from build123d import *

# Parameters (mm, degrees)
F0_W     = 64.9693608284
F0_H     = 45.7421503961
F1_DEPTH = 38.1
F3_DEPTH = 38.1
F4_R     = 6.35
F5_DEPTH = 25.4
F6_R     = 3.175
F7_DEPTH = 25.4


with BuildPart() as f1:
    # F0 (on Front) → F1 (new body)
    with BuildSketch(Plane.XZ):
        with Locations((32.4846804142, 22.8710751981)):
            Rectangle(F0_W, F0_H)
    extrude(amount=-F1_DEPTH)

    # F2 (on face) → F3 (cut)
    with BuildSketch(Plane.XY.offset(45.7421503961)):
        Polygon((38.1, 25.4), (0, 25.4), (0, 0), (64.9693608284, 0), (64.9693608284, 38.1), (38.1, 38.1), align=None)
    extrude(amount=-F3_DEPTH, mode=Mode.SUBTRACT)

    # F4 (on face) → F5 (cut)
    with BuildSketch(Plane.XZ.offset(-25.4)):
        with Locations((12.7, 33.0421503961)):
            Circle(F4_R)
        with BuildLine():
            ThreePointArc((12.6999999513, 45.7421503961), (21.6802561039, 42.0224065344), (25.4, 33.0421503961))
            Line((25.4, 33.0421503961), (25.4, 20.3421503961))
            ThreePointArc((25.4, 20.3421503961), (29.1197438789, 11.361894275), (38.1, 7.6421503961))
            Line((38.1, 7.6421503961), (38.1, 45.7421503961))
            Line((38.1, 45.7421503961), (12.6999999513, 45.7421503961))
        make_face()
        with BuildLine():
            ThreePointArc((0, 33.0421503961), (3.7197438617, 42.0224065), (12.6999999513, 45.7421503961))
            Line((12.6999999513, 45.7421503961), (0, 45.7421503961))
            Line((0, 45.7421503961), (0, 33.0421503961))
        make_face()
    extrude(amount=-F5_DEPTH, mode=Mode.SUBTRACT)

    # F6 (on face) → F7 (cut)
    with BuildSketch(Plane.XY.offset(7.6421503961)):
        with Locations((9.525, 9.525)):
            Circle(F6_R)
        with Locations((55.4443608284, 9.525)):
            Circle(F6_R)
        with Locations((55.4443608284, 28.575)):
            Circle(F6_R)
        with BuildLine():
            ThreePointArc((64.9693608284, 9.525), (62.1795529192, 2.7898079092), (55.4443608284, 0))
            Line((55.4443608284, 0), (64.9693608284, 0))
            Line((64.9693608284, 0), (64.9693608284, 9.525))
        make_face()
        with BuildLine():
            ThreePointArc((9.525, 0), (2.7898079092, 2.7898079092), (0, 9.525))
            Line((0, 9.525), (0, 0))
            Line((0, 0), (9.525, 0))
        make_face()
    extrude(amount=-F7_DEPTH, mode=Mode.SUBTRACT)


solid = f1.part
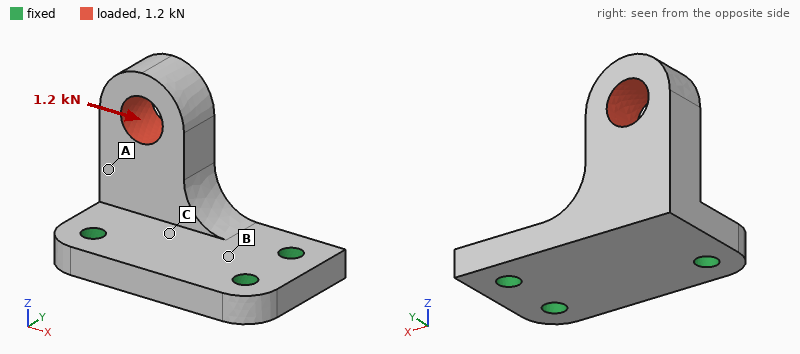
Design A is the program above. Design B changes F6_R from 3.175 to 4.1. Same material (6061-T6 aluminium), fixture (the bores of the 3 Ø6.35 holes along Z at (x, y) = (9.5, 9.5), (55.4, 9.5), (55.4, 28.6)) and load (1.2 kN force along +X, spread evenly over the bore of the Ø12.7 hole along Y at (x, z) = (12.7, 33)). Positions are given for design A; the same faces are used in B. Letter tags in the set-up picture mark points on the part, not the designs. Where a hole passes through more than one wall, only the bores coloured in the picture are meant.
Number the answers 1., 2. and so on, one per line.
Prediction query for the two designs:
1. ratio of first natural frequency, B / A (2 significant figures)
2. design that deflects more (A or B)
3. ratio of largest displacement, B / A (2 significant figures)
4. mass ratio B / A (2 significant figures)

1. 1.0
2. A
3. 0.92
4. 0.98
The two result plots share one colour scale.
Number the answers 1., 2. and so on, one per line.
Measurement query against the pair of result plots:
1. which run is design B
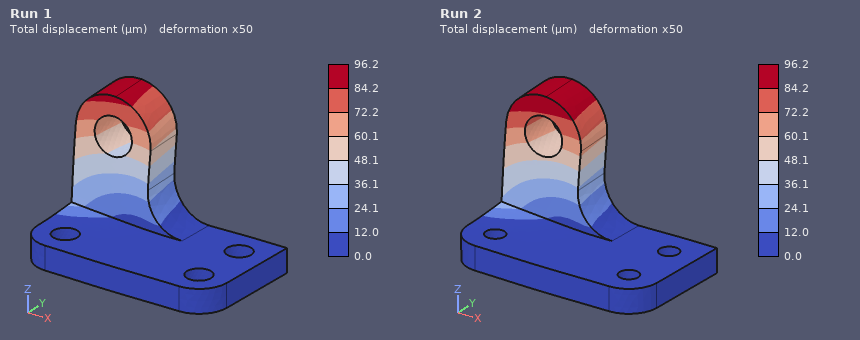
1. Run 1
